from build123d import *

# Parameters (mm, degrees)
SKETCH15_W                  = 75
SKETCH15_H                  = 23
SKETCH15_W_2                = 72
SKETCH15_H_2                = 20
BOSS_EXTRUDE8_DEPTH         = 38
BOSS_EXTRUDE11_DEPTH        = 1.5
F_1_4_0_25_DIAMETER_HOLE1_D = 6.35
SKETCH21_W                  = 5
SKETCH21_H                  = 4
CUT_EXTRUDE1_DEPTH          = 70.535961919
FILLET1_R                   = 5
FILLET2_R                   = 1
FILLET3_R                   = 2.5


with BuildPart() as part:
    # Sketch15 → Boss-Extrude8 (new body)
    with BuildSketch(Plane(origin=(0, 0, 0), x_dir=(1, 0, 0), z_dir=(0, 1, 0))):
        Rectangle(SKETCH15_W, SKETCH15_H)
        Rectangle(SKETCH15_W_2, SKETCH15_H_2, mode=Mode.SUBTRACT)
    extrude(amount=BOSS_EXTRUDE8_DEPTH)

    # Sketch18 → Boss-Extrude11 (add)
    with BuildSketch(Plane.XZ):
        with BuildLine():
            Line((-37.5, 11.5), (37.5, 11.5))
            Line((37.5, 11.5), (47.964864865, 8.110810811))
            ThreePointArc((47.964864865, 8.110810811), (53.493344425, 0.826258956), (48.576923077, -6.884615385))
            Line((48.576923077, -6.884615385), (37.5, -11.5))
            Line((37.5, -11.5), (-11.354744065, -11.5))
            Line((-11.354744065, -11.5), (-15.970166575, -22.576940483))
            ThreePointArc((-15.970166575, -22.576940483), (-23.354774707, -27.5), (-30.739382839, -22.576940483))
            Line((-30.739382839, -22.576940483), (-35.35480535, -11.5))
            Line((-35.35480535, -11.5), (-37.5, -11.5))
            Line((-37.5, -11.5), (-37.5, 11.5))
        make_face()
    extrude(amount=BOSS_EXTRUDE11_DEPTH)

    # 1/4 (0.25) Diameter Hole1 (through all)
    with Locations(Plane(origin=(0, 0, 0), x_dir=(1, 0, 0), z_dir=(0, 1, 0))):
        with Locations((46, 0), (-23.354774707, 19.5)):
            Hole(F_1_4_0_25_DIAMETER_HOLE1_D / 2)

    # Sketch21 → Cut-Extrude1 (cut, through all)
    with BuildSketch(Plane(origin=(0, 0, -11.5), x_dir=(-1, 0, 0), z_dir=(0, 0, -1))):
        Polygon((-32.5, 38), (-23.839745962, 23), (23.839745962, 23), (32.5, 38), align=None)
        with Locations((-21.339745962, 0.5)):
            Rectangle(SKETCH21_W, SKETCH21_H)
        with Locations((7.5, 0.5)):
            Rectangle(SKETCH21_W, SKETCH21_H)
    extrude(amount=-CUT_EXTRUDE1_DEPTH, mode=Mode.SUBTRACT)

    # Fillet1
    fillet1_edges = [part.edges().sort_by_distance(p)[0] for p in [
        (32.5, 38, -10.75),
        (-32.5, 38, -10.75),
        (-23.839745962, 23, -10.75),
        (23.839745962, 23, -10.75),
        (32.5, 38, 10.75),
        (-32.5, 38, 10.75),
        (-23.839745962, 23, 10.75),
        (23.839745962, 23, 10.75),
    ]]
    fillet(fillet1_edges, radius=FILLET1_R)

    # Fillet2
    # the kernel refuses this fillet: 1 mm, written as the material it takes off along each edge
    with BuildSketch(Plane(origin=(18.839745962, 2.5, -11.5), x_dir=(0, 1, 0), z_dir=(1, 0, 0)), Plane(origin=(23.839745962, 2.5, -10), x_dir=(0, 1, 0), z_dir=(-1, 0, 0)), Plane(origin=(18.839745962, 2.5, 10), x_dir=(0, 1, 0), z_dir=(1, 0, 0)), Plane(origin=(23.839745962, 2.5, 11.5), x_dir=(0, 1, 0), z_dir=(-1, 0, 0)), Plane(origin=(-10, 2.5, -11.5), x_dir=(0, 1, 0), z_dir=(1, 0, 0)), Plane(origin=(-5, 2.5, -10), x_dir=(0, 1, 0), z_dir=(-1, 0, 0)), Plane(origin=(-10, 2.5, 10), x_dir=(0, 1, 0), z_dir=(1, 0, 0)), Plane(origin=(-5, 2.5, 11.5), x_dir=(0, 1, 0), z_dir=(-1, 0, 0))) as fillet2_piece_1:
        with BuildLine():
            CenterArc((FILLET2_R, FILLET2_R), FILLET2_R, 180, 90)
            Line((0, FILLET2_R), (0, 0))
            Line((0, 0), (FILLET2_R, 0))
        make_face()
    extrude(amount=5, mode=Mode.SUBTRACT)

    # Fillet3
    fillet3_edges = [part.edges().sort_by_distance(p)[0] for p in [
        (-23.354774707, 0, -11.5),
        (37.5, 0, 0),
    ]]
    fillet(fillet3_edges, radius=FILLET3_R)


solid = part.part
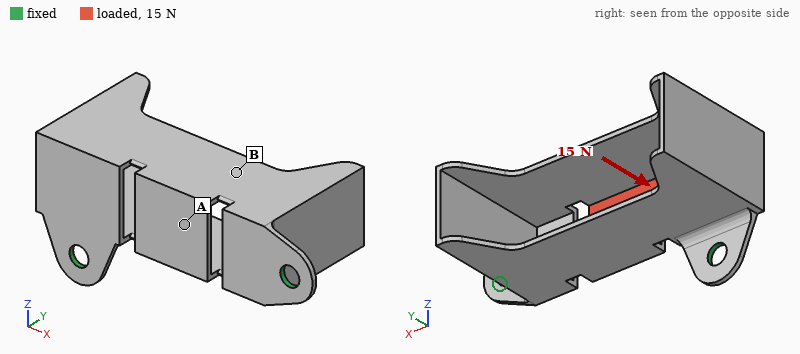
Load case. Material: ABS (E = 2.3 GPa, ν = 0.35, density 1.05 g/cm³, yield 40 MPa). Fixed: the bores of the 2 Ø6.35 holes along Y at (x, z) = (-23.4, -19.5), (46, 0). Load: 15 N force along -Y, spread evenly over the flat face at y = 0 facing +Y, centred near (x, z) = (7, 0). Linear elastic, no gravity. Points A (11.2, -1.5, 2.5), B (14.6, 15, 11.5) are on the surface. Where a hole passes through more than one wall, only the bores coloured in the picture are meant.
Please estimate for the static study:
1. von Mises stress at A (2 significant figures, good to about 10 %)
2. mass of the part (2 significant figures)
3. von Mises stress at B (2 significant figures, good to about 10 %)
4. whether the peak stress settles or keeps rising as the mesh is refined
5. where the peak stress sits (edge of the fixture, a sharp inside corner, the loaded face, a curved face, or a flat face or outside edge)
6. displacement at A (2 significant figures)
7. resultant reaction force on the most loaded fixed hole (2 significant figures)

2.4 MPa
12 g
1.2 MPa
keeps rising
edge of the fixture
0.27 mm
8.5 N
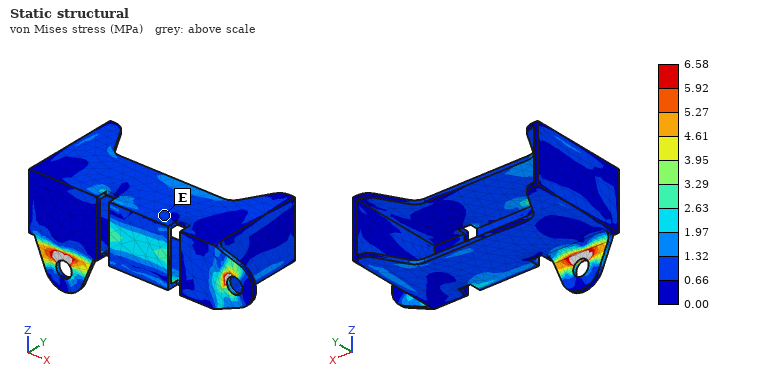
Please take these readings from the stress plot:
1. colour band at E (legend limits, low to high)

0.66 to 1.32 MPa
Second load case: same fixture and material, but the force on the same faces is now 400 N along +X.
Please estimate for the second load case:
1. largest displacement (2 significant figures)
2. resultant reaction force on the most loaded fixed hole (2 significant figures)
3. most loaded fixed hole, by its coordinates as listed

0.69 mm
280 N
(46, 0)
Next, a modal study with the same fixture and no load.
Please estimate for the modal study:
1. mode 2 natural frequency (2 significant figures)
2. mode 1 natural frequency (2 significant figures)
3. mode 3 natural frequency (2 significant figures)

420 Hz
170 Hz
720 Hz
